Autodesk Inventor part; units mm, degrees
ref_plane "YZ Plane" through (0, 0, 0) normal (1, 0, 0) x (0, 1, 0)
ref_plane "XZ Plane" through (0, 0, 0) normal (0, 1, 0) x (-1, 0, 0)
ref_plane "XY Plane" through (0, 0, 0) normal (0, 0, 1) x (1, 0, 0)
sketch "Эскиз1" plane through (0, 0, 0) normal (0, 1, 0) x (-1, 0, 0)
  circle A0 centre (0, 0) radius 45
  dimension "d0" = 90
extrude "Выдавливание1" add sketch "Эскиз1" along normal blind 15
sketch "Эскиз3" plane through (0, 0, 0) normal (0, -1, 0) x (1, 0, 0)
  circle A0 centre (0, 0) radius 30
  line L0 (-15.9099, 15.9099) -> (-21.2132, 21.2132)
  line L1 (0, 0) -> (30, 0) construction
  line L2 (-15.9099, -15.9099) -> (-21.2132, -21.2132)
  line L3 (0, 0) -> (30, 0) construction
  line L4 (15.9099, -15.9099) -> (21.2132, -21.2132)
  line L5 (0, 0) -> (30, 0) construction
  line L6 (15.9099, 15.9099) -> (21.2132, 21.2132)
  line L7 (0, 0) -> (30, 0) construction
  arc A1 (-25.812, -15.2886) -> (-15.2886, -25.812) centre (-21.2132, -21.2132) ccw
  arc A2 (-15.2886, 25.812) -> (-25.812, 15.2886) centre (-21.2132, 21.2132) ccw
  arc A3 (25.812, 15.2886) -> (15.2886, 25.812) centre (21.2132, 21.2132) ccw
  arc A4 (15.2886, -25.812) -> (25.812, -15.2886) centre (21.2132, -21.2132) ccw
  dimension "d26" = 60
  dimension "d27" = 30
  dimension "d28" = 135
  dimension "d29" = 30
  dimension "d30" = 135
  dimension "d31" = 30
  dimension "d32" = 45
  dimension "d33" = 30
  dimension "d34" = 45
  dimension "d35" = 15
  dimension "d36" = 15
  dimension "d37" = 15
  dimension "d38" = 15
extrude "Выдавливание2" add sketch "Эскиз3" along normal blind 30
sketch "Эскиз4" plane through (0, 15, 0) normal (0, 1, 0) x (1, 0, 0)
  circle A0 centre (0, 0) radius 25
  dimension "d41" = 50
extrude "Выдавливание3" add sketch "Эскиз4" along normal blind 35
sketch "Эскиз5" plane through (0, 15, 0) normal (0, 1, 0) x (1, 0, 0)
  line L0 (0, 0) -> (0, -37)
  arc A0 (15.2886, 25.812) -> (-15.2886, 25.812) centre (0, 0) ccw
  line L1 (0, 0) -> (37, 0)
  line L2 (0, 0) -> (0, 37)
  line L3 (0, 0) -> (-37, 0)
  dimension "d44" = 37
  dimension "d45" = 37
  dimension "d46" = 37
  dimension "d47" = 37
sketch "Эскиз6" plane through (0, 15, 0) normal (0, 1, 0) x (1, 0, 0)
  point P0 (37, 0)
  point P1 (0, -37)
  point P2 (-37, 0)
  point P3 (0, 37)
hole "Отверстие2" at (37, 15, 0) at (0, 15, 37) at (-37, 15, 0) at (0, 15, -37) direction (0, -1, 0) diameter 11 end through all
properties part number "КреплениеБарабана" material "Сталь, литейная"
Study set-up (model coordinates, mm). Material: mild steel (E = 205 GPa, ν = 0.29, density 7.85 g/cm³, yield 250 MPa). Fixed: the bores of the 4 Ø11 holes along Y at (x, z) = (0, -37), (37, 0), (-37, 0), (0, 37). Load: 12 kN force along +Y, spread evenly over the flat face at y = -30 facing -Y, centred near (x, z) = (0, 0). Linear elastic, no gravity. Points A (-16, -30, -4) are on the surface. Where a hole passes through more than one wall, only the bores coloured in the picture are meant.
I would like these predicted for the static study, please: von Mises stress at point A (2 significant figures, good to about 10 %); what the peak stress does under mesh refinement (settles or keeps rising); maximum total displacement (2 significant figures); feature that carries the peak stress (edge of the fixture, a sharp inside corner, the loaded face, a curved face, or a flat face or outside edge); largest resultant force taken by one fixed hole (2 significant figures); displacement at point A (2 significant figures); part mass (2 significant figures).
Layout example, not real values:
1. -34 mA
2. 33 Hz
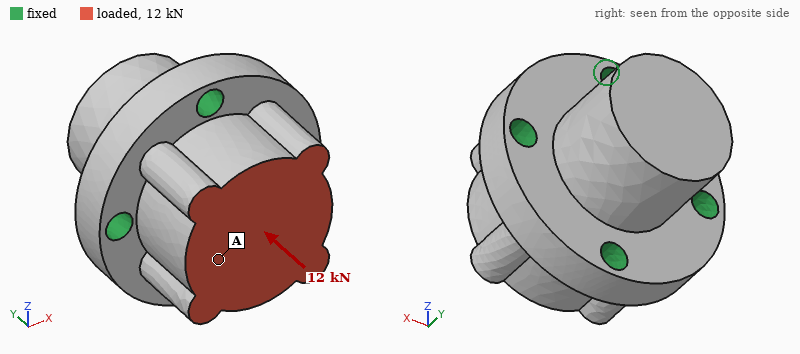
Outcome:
1. 3.6 MPa
2. keeps rising
3. 1.6 µm
4. edge of the fixture
5. 3.1 kN
6. 1.6 µm
7. 2.0 kg
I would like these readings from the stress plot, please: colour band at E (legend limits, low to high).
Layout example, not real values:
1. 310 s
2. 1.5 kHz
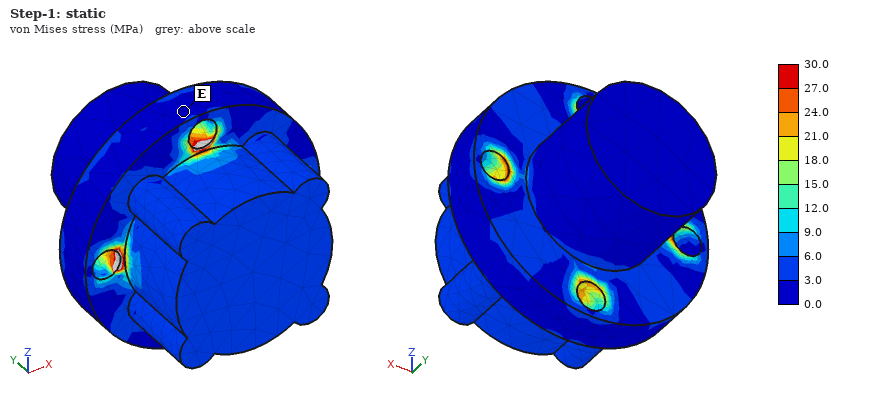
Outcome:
1. 0.0 to 3.0 MPa
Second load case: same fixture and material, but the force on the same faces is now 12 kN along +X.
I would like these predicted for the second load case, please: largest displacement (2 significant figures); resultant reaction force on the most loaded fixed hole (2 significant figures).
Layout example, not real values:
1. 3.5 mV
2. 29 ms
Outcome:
1. 6.4 µm
2. 7.3 kN
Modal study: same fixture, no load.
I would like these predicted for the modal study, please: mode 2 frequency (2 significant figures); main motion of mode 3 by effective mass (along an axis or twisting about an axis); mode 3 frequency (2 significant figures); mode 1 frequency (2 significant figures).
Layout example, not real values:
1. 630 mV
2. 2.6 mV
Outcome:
1. 9700 Hz
2. along Y
3. 12 kHz
4. 9700 Hz
